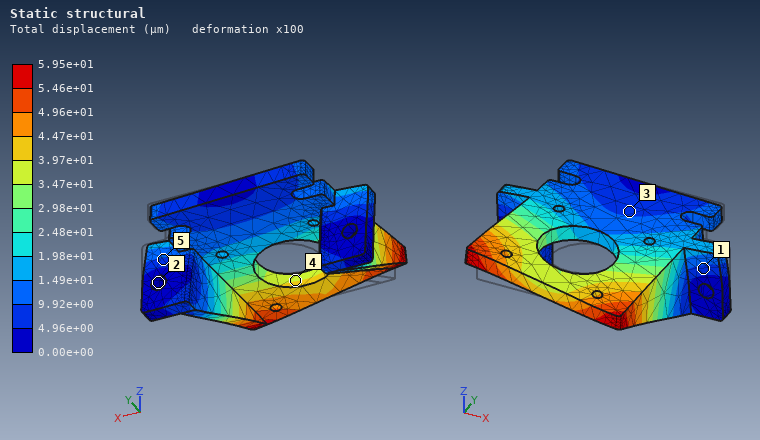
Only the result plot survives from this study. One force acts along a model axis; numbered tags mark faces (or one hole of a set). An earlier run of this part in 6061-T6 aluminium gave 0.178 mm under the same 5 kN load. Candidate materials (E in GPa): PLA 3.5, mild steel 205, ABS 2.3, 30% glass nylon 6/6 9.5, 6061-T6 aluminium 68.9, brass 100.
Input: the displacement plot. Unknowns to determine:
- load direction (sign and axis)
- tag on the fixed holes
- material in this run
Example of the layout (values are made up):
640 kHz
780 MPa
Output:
-X
2
mild steel
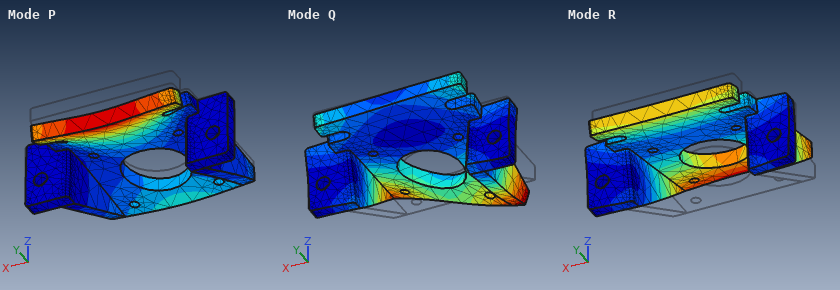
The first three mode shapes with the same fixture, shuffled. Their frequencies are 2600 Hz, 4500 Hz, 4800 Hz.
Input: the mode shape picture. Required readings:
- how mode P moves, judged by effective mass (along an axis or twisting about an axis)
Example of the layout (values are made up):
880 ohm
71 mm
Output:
along Z
